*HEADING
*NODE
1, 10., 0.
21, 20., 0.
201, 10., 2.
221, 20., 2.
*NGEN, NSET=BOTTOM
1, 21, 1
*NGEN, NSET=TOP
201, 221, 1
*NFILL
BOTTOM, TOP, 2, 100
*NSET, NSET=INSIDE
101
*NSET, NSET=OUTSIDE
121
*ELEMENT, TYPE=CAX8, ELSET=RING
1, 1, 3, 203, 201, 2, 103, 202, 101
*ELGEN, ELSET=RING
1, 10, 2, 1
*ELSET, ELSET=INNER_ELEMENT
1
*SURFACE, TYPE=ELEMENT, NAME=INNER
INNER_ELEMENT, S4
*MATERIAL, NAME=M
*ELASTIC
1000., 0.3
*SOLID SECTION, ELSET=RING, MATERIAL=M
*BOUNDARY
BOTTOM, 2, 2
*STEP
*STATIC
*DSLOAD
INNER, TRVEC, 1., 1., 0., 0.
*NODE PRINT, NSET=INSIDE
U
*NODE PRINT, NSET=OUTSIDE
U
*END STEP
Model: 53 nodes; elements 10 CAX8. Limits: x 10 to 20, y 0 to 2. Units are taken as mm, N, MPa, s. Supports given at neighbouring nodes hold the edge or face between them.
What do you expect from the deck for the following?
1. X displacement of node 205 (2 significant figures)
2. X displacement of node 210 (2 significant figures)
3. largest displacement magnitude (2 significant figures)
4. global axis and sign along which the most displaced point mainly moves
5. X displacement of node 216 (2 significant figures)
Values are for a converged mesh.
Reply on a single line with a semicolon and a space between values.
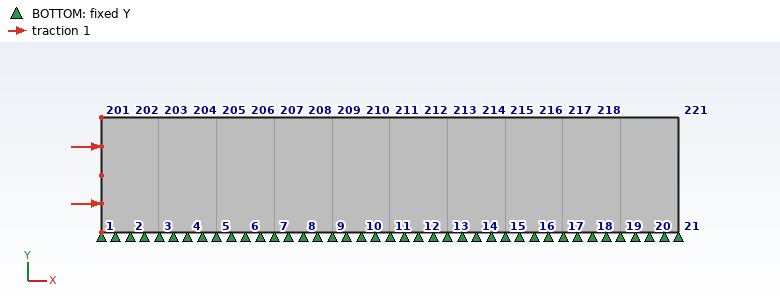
0.017 mm; 0.015 mm; 0.020 mm; +X; 0.014 mm
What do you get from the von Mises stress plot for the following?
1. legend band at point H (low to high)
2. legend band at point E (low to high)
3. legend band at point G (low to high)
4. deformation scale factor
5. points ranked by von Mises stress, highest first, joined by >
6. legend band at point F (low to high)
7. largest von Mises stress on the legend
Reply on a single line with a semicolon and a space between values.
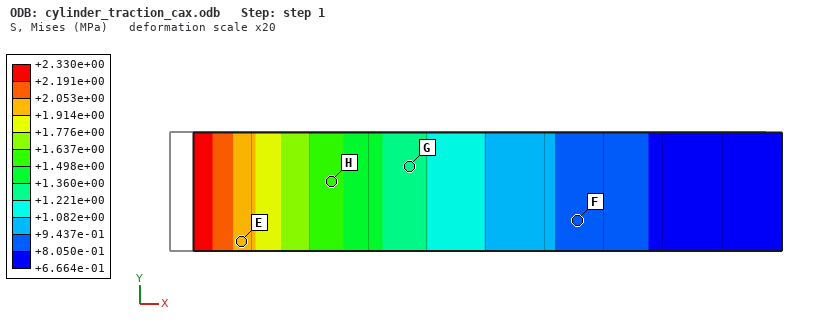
+1.498e+00 to +1.637e+00 MPa; +1.914e+00 to +2.053e+00 MPa; +1.221e+00 to +1.360e+00 MPa; 20; E > H > G > F; +8.050e-01 to +9.437e-01 MPa; +2.330e+00 MPa
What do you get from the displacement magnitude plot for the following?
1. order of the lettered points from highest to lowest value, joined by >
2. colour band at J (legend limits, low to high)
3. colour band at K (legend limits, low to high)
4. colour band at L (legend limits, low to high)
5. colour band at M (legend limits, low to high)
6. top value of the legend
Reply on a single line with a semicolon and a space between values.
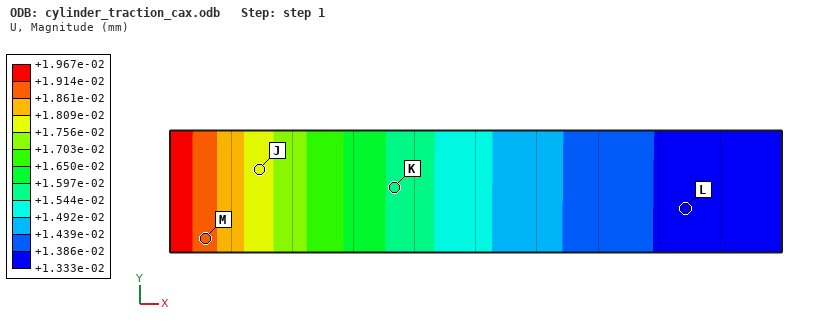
M > J > K > L; +1.756e-02 to +1.809e-02 mm; +1.544e-02 to +1.597e-02 mm; +1.333e-02 to +1.386e-02 mm; +1.861e-02 to +1.914e-02 mm; +1.967e-02 mm
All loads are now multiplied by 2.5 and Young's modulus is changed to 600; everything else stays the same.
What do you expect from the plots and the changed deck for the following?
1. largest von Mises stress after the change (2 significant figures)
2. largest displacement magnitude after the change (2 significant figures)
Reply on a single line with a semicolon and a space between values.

5.8 MPa; 0.082 mm
